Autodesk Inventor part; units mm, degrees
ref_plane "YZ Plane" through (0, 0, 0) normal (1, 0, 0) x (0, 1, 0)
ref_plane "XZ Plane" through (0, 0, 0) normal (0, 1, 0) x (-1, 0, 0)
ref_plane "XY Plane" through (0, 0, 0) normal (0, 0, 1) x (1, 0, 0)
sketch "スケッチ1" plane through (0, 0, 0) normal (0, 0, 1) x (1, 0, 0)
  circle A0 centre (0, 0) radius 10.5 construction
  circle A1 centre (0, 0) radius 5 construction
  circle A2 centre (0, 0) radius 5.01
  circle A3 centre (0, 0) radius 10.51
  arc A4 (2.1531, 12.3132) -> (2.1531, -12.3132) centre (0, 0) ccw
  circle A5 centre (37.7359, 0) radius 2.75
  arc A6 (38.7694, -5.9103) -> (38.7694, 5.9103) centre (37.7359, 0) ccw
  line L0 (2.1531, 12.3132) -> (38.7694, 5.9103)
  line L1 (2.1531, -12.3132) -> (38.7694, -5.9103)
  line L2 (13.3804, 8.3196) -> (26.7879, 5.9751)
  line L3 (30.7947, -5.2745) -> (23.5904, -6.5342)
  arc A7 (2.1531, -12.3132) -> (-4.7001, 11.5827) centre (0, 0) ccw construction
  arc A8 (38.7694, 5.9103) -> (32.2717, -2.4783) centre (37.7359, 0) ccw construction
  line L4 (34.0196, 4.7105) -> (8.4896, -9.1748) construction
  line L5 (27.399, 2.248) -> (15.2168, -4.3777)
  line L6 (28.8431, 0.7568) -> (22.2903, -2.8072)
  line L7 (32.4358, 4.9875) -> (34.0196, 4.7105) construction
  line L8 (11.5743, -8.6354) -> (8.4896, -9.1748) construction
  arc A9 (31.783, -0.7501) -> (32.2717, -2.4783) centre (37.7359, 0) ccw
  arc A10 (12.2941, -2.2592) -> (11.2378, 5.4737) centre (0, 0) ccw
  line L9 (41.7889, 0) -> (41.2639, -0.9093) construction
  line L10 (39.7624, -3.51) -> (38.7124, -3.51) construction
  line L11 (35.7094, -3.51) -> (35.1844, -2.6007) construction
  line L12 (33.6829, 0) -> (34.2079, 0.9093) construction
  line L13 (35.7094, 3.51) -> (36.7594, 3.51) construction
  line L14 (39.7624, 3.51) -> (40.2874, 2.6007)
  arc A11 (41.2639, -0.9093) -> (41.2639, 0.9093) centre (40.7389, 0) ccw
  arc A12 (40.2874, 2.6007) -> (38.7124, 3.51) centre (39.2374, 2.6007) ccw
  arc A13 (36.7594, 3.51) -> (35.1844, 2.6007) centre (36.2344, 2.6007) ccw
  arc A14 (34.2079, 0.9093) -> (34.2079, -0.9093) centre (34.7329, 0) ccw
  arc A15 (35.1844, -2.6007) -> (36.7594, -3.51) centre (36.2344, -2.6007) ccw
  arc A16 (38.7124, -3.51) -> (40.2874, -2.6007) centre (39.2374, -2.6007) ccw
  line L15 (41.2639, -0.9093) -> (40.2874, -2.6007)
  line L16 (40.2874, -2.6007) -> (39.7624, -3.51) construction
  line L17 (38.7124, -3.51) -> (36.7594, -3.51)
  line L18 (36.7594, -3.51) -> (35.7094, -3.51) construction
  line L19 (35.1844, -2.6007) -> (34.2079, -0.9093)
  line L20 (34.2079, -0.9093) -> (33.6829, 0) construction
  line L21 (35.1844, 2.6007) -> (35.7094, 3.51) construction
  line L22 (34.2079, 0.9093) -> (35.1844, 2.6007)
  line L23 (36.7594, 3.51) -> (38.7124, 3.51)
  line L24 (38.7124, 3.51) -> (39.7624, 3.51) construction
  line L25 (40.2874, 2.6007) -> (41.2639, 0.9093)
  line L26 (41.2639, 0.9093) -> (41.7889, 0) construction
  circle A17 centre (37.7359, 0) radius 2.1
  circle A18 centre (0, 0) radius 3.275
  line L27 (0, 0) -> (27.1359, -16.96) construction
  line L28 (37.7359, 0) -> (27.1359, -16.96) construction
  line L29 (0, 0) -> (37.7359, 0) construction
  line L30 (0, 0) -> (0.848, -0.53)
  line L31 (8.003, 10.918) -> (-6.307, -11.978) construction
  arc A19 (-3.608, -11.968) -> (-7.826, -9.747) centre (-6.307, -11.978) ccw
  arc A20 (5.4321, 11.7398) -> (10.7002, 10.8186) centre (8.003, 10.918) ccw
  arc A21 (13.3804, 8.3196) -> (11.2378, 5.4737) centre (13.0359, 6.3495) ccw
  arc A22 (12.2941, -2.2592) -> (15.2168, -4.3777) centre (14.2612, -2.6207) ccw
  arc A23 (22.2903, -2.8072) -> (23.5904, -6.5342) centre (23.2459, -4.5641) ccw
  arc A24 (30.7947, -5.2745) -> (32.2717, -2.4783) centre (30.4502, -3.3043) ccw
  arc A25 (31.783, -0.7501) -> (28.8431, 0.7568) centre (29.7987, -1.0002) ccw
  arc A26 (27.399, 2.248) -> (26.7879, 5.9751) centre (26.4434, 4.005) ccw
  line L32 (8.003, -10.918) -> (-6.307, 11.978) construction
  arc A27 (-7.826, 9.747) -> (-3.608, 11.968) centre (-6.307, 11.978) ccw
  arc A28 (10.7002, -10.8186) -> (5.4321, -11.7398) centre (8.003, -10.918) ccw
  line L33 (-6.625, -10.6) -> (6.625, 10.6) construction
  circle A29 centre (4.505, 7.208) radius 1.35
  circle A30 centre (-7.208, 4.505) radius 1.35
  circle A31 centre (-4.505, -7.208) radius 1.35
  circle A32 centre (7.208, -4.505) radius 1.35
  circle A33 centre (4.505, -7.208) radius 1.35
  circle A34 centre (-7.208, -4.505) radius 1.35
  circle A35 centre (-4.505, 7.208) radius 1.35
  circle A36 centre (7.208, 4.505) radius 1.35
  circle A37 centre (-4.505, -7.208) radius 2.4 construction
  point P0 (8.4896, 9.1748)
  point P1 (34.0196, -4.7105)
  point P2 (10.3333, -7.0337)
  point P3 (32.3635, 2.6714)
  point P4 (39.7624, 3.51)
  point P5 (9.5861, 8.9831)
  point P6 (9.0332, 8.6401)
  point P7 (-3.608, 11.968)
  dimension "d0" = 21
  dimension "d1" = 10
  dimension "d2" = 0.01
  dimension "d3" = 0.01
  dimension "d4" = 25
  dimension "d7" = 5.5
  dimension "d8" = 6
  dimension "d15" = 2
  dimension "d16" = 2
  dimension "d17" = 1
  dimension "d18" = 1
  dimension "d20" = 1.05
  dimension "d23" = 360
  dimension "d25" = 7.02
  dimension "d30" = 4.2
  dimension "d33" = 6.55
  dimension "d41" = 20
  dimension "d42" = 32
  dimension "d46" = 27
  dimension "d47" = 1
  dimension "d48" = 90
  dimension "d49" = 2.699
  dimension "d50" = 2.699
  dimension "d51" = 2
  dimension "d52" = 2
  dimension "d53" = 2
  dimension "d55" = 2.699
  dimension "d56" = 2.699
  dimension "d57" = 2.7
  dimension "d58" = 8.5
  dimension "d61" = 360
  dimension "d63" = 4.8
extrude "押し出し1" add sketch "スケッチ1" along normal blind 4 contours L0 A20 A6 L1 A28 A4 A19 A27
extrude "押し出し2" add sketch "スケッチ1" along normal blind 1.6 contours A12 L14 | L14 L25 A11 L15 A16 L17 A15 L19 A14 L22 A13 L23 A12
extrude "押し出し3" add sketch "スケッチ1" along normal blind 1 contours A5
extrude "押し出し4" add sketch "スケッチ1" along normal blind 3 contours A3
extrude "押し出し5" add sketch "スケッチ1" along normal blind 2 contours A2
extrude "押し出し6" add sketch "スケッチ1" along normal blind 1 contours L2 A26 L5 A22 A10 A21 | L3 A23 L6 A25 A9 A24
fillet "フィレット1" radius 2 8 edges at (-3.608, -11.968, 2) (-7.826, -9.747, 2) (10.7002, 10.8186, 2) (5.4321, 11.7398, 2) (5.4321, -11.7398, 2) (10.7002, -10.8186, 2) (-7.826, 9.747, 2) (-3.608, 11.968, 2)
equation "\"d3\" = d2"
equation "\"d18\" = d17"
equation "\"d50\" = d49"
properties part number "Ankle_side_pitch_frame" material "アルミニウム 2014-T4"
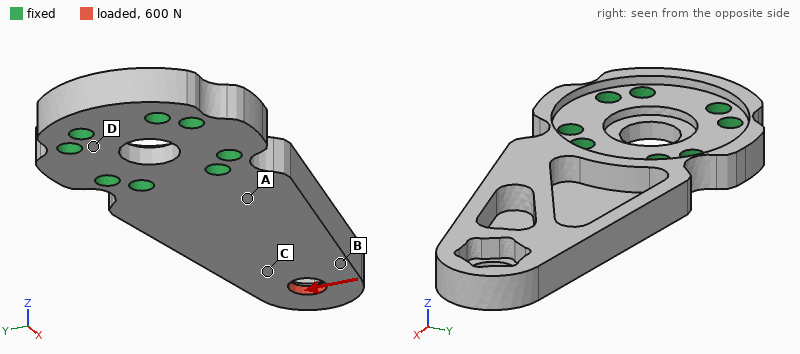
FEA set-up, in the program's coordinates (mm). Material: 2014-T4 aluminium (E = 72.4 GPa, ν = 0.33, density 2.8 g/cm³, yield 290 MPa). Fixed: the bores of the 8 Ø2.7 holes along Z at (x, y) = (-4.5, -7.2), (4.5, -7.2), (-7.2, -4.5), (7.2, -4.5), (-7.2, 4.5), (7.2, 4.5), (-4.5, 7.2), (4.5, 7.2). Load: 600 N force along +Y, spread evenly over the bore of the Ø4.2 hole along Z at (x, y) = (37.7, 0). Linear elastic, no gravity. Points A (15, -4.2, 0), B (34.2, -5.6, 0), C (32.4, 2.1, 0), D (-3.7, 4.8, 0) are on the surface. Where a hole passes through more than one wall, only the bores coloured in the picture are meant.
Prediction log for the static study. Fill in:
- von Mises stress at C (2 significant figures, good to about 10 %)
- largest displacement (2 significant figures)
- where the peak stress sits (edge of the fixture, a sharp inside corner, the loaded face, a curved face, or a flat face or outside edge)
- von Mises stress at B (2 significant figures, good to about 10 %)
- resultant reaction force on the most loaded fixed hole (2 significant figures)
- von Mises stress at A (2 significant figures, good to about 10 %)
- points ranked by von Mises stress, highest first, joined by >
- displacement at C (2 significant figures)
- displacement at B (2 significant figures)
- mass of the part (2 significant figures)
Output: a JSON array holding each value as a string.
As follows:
["50 MPa", "0.14 mm", "a curved face", "39 MPa", "870 N", "79 MPa", "A > C > B > D", "0.087 mm", "0.090 mm", "7.1 g"]
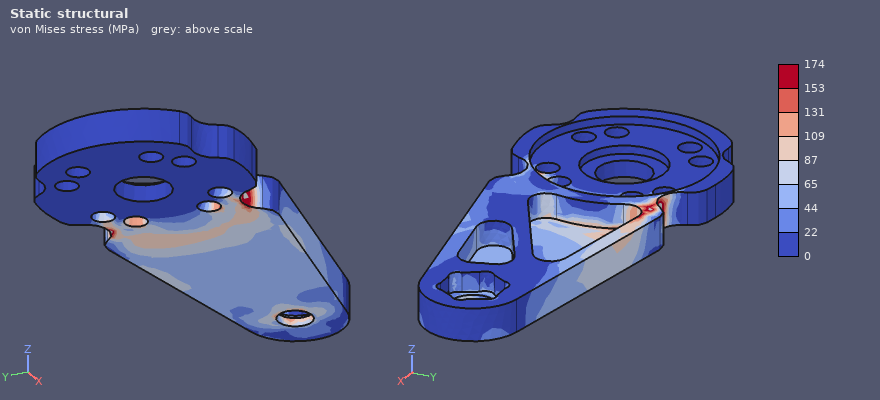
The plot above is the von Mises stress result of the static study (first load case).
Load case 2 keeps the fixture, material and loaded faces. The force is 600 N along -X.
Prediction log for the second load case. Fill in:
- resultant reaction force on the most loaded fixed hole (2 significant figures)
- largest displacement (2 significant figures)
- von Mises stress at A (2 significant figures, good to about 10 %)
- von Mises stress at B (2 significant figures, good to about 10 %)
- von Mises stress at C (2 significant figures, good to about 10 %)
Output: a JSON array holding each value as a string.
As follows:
["240 N", "0.10 mm", "32 MPa", "38 MPa", "40 MPa"]
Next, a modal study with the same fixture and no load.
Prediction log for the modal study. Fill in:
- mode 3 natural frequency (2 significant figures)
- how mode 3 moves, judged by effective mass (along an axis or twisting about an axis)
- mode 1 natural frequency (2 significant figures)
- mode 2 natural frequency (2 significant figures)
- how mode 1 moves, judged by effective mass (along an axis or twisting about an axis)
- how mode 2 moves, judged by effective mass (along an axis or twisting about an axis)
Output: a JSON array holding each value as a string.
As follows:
["11 kHz", "along Y", "2600 Hz", "9200 Hz", "along Z", "along Y"]
